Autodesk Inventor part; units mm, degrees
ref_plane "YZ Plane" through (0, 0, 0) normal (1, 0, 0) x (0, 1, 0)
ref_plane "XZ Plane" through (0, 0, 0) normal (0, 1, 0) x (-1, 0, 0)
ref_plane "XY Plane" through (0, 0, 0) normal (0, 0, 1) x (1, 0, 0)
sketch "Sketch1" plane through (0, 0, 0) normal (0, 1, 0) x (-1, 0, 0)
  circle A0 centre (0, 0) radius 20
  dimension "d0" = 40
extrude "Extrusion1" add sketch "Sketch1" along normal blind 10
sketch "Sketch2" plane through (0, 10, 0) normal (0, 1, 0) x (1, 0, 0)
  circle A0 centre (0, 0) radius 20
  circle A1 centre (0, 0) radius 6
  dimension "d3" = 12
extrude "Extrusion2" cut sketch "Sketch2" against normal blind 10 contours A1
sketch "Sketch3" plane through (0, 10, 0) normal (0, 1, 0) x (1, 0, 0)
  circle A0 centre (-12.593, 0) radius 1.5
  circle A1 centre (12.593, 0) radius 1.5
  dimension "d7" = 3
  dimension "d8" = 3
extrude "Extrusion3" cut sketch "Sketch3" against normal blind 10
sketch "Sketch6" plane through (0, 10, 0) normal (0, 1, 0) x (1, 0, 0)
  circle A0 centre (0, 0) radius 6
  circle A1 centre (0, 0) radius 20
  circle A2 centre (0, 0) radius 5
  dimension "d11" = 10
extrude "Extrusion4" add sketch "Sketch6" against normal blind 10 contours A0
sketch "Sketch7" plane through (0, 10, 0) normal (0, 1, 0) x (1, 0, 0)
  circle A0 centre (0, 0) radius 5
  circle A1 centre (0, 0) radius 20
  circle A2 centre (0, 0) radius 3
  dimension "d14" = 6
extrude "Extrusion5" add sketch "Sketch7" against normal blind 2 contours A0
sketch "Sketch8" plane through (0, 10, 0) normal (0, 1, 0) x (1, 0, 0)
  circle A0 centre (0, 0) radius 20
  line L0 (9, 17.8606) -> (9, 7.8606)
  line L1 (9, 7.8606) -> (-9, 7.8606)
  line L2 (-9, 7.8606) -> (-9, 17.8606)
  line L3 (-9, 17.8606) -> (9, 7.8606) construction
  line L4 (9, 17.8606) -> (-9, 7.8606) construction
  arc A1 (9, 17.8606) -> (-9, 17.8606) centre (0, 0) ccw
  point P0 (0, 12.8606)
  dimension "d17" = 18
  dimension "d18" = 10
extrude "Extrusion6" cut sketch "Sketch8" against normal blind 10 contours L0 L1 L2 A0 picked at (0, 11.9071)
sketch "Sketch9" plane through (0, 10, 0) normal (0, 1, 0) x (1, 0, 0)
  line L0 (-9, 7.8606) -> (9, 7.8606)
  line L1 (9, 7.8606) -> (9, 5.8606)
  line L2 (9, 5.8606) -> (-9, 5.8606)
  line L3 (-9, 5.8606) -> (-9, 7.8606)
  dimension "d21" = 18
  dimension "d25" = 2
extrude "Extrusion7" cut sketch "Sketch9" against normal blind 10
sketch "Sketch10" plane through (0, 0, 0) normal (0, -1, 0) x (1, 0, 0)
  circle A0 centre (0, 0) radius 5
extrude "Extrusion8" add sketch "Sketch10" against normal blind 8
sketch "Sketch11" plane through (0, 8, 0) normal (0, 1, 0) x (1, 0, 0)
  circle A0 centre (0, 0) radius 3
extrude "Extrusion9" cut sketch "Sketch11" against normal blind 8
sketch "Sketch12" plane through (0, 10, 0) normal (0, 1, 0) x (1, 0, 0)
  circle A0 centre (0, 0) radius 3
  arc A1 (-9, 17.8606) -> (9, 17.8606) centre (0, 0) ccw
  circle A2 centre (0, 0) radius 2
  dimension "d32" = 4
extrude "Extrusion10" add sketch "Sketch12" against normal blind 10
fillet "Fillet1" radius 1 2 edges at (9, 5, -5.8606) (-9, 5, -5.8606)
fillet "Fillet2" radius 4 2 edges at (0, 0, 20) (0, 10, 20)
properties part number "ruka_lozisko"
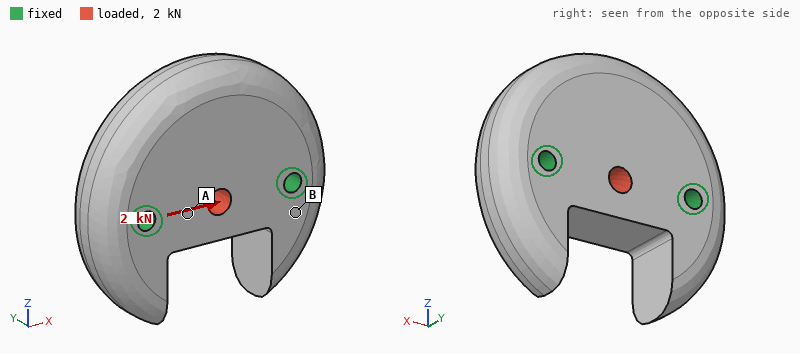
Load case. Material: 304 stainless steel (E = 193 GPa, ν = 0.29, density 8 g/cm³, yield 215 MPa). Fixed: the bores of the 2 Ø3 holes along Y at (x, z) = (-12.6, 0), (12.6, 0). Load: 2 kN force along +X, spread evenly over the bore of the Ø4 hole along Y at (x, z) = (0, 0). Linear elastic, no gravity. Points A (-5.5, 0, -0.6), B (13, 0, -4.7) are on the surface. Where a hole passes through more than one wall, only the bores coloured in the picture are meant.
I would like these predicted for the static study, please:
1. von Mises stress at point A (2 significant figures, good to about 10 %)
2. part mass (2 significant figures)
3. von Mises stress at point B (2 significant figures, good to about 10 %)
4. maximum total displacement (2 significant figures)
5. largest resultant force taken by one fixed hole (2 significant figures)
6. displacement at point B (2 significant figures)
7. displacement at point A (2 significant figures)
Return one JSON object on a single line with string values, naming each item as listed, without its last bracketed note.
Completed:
{"von Mises stress at point A": "14 MPa", "part mass": "74 g", "von Mises stress at point B": "3.5 MPa", "maximum total displacement": "0.72 µm", "largest resultant force taken by one fixed hole": "1.0 kN", "displacement at point B": "0.18 µm", "displacement at point A": "0.41 µm"}
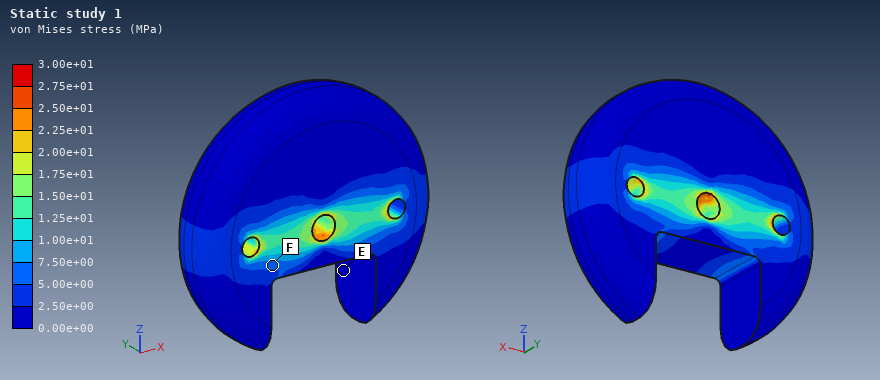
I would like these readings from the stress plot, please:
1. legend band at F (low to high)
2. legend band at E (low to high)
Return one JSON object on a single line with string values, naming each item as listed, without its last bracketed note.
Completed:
{"legend band at F": "5.00e+00 to 7.50e+00 MPa", "legend band at E": "0.00e+00 to 2.50e+00 MPa"}
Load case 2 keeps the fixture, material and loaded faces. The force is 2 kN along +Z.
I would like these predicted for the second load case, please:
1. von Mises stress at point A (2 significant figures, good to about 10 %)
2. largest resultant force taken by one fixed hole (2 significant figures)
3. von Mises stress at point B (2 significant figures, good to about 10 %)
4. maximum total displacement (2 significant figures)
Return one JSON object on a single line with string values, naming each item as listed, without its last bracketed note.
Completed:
{"von Mises stress at point A": "10 MPa", "largest resultant force taken by one fixed hole": "1.0 kN", "von Mises stress at point B": "4.7 MPa", "maximum total displacement": "1.6 µm"}
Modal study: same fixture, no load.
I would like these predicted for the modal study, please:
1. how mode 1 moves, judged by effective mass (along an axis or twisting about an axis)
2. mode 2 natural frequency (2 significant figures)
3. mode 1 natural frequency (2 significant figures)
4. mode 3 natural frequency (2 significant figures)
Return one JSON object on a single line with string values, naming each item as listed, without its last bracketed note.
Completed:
{"how mode 1 moves, judged by effective mass": "along Y", "mode 2 natural frequency": "32 kHz", "mode 1 natural frequency": "17 kHz", "mode 3 natural frequency": "32 kHz"}
